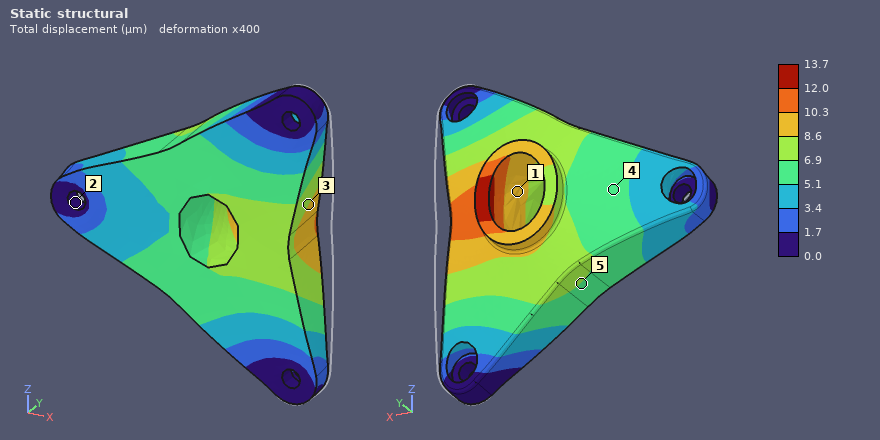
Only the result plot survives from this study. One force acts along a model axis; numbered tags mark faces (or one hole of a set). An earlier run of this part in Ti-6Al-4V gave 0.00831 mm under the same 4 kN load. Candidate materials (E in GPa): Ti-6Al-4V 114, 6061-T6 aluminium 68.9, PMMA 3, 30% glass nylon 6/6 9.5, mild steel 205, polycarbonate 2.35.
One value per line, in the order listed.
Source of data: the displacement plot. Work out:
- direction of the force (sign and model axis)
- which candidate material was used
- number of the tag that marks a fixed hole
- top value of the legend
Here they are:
-X
6061-T6 aluminium
2
13.7 µm
